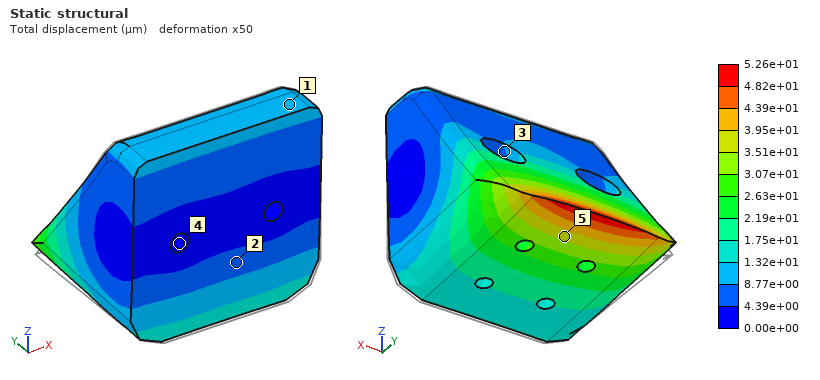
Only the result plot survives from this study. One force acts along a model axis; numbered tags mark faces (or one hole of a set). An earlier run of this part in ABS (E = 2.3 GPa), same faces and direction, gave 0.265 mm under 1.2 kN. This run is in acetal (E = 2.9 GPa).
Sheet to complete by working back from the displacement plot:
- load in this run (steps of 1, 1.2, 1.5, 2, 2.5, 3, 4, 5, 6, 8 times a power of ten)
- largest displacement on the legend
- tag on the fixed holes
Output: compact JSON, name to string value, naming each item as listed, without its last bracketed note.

{"load in this run": "300 N", "largest displacement on the legend": "5.26e+01 µm", "tag on the fixed holes": "4"}
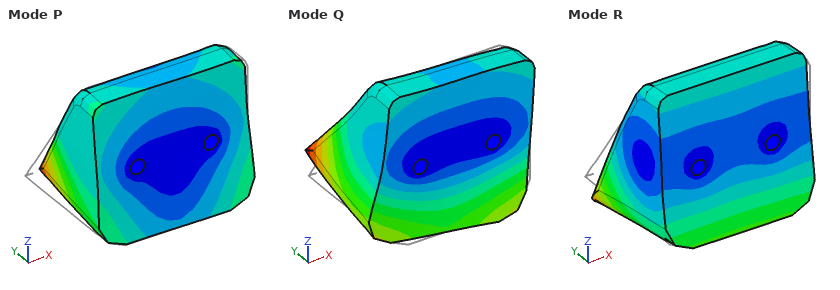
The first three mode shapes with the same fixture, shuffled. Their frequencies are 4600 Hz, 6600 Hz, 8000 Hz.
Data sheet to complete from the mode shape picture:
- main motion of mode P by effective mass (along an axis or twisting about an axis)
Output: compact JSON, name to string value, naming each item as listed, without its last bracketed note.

{"main motion of mode P by effective mass": "along X"}
